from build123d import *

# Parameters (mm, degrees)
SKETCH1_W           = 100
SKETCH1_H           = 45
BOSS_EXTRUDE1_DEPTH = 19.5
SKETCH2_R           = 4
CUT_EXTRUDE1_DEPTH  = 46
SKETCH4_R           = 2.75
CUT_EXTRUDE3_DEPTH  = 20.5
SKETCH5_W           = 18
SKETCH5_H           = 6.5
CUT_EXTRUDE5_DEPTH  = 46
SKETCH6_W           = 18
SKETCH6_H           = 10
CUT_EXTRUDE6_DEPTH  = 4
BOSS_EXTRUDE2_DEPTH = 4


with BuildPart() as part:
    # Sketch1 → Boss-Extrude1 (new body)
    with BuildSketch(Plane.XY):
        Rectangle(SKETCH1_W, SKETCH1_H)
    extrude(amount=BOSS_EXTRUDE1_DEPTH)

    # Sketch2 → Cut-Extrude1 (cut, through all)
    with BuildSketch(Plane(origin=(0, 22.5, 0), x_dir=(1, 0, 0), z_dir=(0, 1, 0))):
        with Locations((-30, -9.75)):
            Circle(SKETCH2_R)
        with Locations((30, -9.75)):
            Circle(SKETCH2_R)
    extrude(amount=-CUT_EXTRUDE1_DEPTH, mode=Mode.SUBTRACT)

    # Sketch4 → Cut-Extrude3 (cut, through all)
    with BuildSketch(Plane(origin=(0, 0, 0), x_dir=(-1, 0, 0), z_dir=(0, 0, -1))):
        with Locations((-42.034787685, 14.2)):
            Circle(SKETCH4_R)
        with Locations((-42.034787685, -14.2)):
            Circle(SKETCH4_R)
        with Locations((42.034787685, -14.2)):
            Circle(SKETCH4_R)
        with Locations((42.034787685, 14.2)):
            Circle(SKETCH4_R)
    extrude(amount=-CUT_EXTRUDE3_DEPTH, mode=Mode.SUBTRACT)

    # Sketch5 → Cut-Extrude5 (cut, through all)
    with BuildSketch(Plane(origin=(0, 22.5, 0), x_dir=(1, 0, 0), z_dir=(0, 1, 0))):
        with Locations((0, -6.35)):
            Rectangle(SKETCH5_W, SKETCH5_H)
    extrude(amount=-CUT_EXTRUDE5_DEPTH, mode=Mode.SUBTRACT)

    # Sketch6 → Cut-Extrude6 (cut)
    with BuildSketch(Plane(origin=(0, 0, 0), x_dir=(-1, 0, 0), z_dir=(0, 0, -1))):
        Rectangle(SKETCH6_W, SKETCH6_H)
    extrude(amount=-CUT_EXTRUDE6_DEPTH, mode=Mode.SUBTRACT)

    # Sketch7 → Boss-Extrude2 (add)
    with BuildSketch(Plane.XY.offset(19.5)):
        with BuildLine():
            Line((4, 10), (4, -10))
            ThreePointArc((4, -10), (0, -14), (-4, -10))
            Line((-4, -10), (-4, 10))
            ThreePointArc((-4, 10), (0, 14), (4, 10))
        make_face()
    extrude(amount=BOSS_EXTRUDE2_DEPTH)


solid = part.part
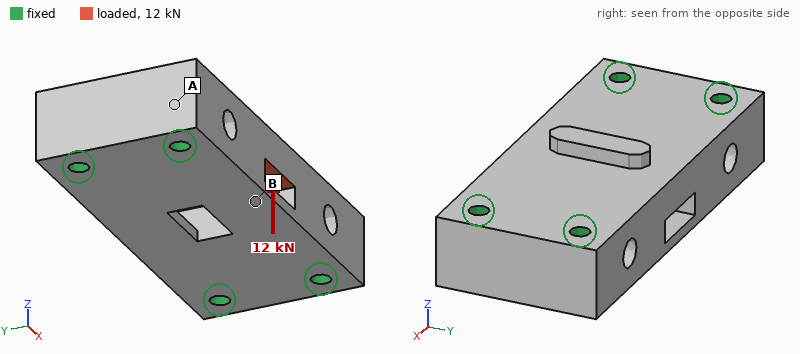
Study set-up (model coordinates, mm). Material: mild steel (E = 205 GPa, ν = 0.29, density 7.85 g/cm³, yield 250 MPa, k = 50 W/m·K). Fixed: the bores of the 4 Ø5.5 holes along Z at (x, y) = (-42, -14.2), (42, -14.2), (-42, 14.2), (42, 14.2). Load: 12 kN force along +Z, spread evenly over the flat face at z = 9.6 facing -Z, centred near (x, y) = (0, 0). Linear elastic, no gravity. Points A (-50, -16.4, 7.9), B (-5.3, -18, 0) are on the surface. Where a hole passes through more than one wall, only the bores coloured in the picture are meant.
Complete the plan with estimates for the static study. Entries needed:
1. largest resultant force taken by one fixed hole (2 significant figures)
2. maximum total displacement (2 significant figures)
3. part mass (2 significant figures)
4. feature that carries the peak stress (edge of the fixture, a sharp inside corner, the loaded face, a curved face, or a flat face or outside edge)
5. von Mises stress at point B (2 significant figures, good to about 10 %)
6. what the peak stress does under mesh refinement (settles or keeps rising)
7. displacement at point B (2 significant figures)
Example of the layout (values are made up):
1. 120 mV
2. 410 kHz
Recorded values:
1. 3.1 kN
2. 16 µm
3. 600 g
4. edge of the fixture
5. 38 MPa
6. keeps rising
7. 12 µm
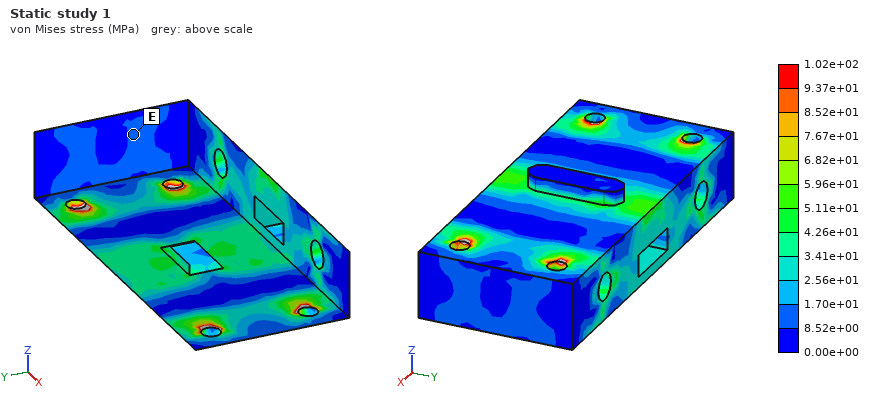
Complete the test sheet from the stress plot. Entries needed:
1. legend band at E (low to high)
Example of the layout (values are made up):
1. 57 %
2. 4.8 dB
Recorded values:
1. 8.52e+00 to 1.70e+01 MPa
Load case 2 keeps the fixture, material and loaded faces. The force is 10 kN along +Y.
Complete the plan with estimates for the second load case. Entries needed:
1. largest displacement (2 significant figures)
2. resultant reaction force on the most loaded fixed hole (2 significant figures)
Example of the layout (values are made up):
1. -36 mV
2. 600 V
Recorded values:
1. 7.2 µm
2. 3.9 kN
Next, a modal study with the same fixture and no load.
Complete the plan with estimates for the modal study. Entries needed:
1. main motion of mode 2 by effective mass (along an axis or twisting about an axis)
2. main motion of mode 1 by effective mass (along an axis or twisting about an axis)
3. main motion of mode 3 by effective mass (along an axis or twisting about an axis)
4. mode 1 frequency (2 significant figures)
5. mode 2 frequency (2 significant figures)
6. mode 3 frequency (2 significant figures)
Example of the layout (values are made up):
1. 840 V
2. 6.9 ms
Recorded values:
1. along Y
2. along Z
3. along Y
4. 9800 Hz
5. 14 kHz
6. 15 kHz
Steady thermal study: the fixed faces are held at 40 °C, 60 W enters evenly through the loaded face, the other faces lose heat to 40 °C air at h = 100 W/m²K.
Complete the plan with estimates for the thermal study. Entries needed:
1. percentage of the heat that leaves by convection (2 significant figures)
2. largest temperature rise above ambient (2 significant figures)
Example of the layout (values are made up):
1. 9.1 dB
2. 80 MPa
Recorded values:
1. 30 %
2. 34 K
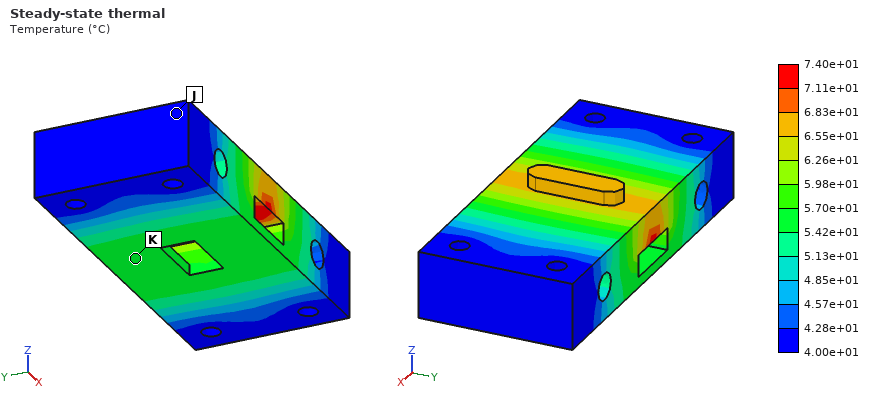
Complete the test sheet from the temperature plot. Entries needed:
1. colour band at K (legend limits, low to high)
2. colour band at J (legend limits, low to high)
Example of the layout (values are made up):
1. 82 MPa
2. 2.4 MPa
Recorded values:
1. 5.42e+01 to 5.70e+01 °C
2. 4.00e+01 to 4.28e+01 °C
